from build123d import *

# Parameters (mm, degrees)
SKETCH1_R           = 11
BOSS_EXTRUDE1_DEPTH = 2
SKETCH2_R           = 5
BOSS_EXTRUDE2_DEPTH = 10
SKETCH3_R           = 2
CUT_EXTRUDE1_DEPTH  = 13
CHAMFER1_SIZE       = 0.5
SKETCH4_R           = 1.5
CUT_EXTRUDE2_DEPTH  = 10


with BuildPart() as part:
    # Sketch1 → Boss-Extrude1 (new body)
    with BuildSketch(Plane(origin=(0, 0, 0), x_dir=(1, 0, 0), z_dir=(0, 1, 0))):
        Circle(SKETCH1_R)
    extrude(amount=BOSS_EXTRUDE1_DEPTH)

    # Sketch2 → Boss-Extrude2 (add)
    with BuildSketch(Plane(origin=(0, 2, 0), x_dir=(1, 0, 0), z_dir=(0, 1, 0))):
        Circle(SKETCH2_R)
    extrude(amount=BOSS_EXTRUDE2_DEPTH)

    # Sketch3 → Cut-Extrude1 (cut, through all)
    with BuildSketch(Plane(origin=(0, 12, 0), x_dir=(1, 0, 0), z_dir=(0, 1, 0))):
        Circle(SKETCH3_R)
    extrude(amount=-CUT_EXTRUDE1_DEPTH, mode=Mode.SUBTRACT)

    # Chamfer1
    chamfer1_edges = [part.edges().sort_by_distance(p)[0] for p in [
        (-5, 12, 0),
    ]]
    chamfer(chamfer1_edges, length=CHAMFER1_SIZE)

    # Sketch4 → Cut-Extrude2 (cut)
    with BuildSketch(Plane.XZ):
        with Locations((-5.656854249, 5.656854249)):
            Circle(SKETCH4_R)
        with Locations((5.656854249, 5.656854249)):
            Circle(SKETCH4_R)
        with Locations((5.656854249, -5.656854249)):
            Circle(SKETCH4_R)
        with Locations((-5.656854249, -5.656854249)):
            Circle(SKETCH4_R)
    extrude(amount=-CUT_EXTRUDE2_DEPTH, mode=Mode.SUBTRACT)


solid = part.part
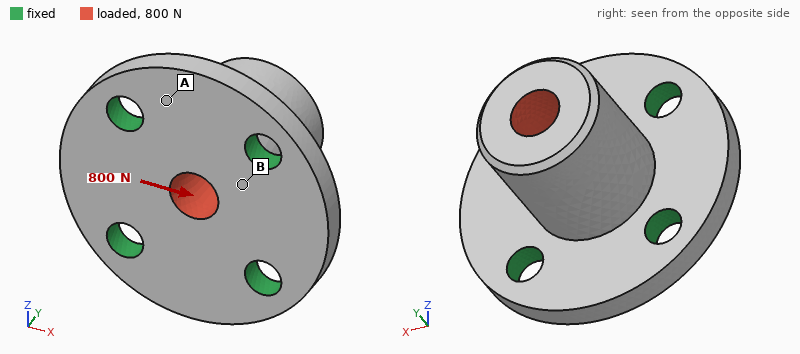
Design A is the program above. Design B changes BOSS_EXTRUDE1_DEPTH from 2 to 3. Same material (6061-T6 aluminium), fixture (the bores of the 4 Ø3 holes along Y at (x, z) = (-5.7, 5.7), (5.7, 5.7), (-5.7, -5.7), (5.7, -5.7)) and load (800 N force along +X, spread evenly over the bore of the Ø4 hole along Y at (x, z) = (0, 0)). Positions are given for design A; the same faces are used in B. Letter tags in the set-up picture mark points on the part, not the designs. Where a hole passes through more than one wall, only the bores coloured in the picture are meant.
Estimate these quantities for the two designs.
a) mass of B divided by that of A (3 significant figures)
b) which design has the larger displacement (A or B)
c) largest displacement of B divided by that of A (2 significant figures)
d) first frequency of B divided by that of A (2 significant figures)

1.20
A
0.57
1.3
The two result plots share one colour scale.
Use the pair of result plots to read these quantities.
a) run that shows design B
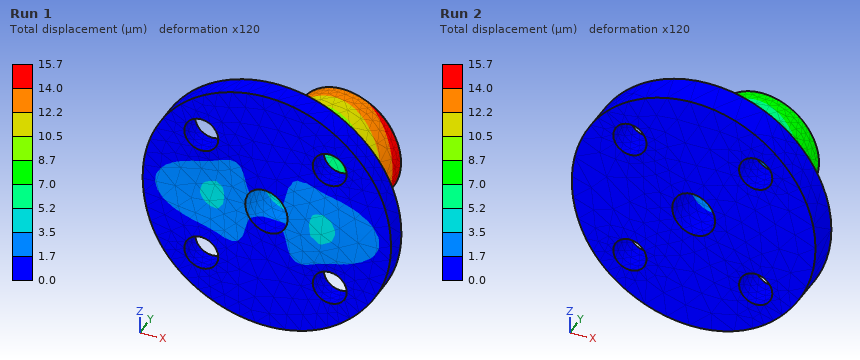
Run 2
